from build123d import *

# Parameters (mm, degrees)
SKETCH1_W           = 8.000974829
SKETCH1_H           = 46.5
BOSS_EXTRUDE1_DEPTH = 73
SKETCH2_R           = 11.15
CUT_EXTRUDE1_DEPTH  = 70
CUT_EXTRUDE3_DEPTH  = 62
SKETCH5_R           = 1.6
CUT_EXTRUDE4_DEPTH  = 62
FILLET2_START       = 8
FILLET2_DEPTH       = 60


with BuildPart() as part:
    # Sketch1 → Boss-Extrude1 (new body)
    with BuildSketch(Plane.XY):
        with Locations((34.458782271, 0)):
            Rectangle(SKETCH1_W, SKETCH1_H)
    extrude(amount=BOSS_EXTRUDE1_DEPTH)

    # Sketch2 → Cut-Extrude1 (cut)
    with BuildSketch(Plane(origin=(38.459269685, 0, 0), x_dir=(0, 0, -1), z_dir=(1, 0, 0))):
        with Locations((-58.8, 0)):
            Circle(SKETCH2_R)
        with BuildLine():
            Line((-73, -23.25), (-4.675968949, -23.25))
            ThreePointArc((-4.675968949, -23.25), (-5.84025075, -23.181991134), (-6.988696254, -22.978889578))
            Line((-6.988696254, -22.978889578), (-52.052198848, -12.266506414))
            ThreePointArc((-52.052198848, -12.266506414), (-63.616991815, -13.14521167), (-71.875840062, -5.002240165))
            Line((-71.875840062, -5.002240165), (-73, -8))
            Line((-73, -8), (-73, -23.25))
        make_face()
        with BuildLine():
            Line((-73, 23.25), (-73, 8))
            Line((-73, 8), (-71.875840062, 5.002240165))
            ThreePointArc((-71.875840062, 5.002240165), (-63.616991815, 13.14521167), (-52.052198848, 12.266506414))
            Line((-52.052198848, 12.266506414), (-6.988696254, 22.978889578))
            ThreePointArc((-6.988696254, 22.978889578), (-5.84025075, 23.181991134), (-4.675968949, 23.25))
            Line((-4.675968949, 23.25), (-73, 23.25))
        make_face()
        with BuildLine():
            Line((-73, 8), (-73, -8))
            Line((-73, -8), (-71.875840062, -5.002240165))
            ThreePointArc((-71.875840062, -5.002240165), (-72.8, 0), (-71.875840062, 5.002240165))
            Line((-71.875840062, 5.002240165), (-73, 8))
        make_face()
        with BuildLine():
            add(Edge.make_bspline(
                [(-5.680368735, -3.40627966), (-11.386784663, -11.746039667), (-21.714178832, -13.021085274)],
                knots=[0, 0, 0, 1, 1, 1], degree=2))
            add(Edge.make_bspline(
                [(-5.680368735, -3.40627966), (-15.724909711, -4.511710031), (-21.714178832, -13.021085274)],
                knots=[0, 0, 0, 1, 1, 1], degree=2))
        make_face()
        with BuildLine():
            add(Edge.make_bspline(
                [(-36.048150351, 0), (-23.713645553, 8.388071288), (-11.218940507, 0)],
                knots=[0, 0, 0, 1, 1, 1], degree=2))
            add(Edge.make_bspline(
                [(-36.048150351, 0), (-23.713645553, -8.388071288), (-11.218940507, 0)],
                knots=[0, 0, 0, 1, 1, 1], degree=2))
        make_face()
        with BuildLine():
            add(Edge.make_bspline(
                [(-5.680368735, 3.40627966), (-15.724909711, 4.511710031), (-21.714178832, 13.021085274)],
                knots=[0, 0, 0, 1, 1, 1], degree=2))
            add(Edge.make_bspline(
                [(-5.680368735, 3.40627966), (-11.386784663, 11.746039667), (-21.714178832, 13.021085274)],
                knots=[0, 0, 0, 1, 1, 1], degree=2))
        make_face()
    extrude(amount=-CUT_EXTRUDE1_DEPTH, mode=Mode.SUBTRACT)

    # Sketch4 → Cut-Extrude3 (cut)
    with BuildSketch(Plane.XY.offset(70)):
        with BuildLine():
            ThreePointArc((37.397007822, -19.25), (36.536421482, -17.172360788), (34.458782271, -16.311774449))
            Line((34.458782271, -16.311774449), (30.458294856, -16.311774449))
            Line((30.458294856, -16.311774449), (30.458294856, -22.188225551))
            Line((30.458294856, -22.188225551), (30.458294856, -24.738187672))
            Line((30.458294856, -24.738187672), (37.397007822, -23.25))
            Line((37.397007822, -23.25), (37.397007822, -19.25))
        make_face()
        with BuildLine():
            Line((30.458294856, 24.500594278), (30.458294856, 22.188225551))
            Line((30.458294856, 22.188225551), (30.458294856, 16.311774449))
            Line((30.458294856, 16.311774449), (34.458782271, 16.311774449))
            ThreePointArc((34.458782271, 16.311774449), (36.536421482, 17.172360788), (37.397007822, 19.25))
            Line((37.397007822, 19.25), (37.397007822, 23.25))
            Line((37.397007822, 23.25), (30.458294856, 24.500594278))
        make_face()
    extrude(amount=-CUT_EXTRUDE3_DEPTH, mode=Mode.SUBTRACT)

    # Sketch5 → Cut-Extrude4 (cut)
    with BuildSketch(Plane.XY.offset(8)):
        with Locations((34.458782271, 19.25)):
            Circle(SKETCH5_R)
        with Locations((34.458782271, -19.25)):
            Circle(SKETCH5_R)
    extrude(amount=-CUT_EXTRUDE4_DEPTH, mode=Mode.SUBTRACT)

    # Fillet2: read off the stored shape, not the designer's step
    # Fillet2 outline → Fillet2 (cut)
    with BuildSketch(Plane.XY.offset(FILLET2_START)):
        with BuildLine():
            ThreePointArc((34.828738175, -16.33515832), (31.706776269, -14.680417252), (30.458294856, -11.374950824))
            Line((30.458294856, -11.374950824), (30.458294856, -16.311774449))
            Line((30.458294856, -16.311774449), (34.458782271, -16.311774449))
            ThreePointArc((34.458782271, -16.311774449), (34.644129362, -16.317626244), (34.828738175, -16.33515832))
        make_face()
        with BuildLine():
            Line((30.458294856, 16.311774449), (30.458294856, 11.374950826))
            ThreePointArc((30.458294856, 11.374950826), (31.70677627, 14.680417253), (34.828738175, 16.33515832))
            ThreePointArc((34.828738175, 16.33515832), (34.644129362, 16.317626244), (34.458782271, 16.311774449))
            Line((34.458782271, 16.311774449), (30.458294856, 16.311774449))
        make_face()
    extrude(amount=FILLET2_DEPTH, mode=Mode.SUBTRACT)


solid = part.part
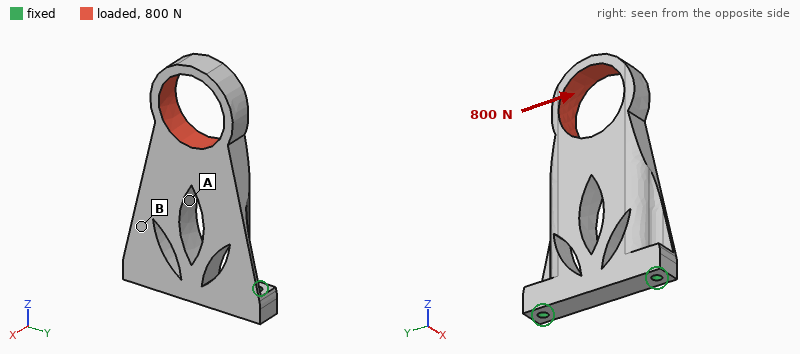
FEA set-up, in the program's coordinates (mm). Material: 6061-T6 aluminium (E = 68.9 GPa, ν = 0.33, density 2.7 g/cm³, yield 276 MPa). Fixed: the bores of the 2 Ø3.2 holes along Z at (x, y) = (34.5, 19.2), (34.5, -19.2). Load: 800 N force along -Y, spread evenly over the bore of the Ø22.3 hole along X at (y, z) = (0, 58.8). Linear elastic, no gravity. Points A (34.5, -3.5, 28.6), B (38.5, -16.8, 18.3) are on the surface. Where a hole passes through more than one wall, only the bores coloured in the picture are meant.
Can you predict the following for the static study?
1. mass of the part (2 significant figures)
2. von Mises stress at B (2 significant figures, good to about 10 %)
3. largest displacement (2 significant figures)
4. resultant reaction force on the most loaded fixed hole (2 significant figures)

34 g
49 MPa
0.18 mm
1.3 kN
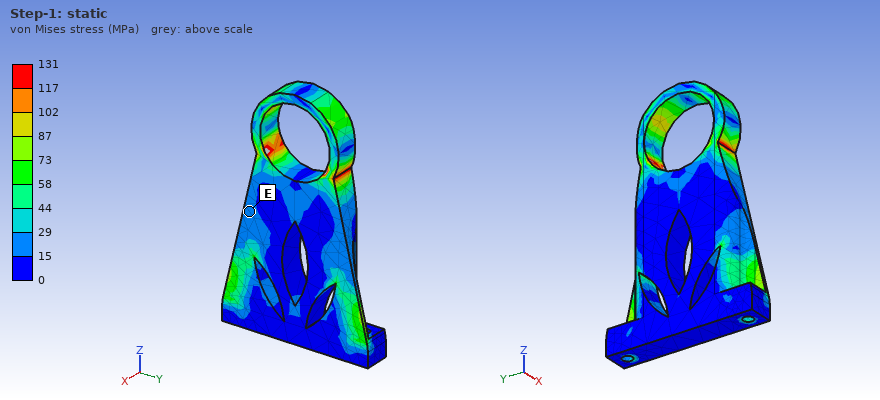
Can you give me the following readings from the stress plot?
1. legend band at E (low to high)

15 to 29 MPa
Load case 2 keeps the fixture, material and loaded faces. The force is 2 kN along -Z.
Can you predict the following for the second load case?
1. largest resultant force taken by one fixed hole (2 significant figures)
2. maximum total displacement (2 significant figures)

1.0 kN
95 µm
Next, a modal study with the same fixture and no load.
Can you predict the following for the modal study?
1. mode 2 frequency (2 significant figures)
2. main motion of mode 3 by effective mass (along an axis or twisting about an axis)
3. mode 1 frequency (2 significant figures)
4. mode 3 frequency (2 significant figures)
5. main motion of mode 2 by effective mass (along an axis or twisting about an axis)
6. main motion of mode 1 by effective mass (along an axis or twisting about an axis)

4900 Hz
twisting about Z
1400 Hz
5800 Hz
along Y
along X
